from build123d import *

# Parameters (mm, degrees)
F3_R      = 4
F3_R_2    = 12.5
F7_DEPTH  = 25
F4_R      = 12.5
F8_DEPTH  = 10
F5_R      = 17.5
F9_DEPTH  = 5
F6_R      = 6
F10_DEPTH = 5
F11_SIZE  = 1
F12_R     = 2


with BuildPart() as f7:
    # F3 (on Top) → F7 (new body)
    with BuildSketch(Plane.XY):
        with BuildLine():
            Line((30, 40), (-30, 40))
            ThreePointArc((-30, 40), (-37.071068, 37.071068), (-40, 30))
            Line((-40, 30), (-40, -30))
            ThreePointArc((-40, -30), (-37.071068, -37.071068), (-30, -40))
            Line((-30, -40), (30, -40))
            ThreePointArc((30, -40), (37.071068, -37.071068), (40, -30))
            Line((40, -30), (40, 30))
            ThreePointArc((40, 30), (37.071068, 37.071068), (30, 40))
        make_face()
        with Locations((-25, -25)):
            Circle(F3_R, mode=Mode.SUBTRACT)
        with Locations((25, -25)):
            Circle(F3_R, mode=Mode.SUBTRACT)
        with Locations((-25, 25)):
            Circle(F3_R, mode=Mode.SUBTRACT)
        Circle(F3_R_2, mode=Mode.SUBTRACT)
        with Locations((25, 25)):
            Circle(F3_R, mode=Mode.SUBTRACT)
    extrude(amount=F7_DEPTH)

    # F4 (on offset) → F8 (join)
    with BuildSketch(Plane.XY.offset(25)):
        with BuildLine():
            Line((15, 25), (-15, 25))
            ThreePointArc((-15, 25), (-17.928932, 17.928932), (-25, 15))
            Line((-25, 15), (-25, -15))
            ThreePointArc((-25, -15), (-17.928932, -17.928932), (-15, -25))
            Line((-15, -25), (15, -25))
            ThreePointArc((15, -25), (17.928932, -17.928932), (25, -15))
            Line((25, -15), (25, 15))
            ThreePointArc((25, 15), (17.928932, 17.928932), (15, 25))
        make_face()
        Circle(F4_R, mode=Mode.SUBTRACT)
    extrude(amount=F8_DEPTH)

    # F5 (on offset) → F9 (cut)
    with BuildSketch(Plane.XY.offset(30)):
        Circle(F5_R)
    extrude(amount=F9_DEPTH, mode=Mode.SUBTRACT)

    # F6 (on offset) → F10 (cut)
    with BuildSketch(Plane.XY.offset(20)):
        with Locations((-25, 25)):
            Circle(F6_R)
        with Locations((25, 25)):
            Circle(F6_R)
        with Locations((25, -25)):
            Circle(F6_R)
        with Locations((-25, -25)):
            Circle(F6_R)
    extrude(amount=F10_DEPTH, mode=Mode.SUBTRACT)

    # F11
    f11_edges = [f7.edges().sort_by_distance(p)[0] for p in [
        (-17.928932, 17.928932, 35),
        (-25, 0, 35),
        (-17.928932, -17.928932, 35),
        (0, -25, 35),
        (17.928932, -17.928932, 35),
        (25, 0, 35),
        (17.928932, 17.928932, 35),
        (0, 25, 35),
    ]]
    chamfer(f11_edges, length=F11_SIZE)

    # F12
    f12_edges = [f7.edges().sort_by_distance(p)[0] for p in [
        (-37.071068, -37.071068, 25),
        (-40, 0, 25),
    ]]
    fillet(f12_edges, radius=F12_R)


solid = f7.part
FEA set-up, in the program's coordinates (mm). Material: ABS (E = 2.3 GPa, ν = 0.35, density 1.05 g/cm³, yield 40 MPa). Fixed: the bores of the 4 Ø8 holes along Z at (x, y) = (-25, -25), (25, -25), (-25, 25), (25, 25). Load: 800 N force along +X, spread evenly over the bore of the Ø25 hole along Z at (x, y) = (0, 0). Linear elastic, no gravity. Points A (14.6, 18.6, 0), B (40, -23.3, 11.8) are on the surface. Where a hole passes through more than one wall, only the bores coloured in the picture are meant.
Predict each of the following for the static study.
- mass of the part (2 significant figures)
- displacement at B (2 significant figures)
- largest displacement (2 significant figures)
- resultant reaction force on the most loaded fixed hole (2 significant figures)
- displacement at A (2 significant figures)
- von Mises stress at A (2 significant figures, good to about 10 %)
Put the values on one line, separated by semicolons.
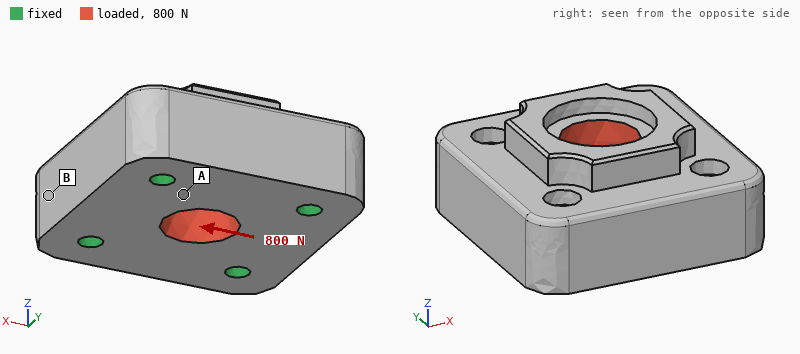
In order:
160 g; 1.7 µm; 7.5 µm; 210 N; 1.9 µm; 0.37 MPa
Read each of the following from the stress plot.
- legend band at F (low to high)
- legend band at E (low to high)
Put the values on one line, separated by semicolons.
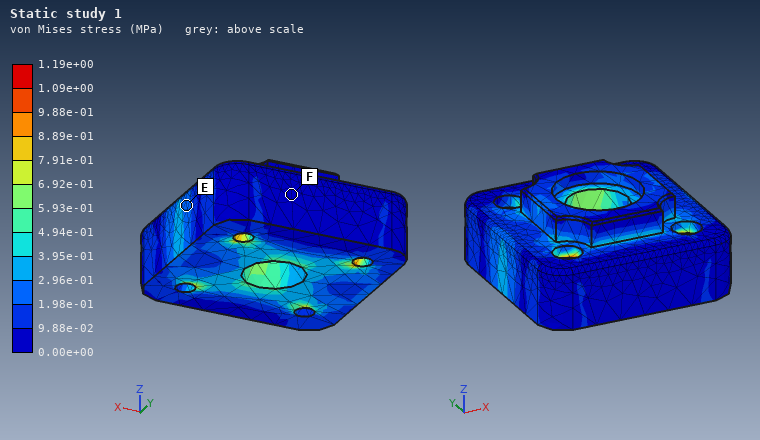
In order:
0.00e+00 to 9.88e-02 MPa; 1.98e-01 to 2.96e-01 MPa
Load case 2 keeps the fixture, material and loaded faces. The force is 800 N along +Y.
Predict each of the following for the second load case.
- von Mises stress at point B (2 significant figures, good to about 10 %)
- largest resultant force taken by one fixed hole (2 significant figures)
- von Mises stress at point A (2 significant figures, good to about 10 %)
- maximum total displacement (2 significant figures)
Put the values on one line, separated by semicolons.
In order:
0.088 MPa; 210 N; 0.36 MPa; 7.4 µm
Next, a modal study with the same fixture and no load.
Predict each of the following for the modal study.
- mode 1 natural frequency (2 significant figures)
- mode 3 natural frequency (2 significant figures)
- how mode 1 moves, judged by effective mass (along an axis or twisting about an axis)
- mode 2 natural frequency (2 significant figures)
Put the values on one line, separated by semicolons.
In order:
5900 Hz; 6500 Hz; along Z; 6300 Hz
